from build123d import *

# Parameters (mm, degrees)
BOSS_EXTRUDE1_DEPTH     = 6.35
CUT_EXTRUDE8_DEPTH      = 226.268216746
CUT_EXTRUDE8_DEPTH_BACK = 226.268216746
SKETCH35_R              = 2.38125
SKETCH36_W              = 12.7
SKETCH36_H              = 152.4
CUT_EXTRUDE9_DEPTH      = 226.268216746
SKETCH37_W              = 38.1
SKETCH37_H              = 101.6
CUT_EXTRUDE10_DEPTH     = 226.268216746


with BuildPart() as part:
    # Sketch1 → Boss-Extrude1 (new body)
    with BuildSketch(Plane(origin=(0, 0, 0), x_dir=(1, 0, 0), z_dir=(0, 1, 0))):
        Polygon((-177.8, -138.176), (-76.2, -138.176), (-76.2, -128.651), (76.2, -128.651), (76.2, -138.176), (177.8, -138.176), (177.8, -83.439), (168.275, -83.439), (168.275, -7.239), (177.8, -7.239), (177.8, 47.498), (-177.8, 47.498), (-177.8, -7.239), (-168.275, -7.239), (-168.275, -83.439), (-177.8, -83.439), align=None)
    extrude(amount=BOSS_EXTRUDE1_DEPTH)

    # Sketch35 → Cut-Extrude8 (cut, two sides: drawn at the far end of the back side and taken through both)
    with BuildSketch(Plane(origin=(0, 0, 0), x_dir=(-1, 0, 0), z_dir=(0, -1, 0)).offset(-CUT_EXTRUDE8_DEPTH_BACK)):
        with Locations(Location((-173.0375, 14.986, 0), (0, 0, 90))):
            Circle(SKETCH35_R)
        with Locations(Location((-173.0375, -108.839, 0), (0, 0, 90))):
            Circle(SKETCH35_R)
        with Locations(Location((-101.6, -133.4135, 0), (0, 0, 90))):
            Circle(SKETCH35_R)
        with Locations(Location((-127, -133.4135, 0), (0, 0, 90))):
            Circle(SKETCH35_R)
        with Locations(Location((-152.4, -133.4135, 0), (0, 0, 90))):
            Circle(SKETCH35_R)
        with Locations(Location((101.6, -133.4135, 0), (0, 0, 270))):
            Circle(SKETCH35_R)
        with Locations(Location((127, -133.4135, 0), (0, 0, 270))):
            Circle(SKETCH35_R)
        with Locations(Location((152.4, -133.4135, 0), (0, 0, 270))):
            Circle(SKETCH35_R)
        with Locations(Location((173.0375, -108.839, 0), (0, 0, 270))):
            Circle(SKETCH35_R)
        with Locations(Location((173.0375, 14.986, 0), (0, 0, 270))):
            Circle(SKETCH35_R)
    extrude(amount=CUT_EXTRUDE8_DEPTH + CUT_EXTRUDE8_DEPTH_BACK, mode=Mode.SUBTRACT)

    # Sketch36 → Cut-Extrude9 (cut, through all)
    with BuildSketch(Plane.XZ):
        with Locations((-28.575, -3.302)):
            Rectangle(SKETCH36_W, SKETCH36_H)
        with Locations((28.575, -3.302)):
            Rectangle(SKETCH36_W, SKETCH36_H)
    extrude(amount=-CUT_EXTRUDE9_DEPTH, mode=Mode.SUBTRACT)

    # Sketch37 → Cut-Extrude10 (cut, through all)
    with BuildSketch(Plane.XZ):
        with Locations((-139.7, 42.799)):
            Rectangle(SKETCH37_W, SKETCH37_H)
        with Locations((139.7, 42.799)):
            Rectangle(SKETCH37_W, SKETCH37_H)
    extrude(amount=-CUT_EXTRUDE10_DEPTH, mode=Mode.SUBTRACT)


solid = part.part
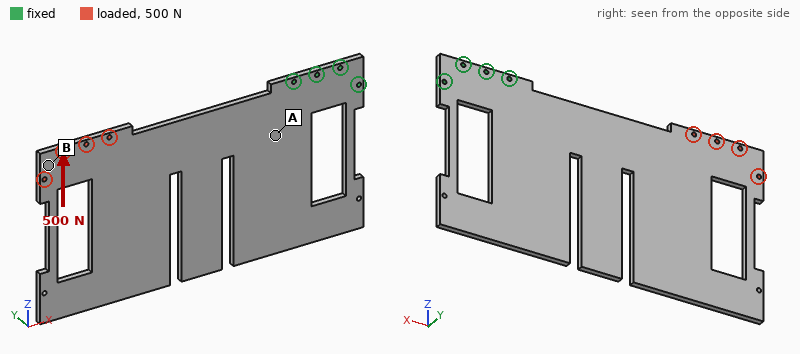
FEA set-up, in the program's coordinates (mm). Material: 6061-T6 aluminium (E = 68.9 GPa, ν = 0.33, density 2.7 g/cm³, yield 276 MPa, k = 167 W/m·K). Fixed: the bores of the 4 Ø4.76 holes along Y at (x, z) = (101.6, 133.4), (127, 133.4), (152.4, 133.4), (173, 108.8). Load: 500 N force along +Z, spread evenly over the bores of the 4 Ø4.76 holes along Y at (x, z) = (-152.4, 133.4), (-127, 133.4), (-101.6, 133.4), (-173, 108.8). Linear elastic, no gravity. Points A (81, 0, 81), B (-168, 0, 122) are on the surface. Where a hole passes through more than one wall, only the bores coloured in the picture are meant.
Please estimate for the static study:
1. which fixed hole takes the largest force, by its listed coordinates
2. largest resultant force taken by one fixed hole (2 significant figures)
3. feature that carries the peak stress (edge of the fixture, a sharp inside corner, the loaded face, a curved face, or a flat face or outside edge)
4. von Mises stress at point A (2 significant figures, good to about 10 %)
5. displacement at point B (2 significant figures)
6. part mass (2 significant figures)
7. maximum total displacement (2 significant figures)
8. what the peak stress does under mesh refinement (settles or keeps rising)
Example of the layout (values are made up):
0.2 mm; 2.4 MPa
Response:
(101.6, 133.4); 2.9 kN; edge of the fixture; 12 MPa; 0.44 mm; 890 g; 0.55 mm; keeps rising
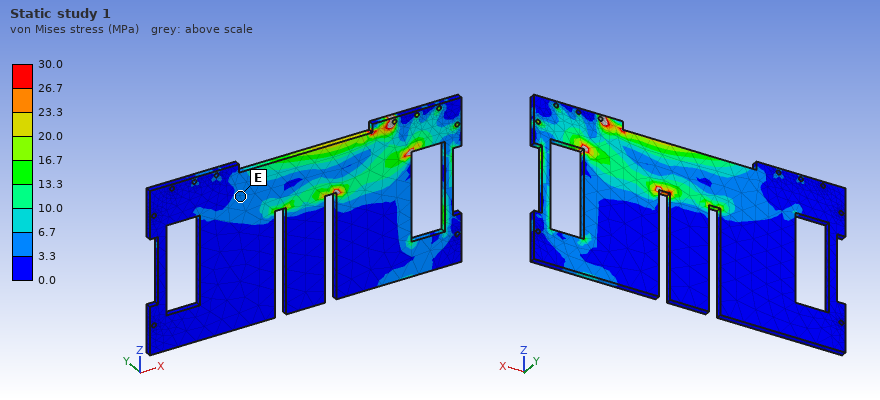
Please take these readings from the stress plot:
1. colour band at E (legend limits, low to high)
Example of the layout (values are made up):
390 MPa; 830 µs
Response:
3.3 to 6.7 MPa
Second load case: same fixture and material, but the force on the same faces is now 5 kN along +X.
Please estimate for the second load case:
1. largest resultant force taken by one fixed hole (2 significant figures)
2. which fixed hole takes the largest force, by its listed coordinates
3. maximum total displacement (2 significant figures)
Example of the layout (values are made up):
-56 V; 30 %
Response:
3.2 kN; (101.6, 133.4); 0.68 mm
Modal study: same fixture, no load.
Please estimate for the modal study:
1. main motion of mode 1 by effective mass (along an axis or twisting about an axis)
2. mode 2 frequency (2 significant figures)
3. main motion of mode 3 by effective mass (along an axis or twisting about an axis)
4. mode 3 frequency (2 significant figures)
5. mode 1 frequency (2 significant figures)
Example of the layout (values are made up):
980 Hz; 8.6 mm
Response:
along Y; 100 Hz; along Y; 160 Hz; 39 Hz
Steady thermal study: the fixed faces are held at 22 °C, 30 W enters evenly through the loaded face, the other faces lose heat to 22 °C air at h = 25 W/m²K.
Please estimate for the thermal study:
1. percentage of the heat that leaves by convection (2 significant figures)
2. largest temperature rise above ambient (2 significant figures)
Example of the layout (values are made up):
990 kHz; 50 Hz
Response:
90 %; 40 K
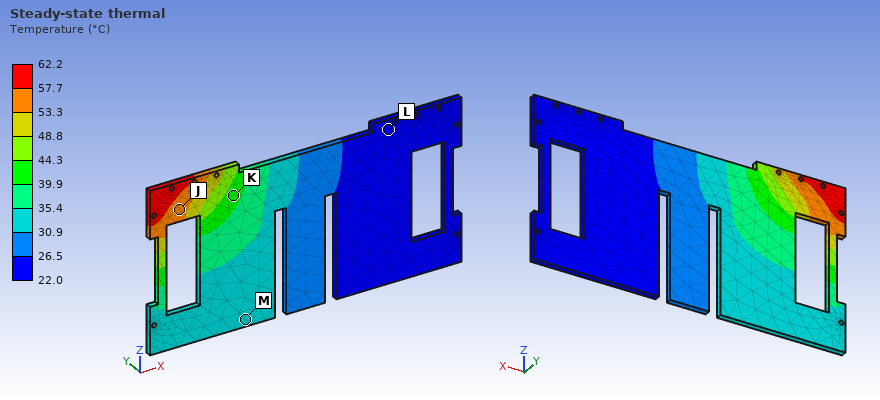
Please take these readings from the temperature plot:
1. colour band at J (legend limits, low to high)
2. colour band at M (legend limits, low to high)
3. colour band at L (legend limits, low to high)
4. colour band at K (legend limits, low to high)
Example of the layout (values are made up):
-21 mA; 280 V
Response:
53.3 to 57.7 °C; 30.9 to 35.4 °C; 22.0 to 26.5 °C; 39.9 to 44.3 °C
